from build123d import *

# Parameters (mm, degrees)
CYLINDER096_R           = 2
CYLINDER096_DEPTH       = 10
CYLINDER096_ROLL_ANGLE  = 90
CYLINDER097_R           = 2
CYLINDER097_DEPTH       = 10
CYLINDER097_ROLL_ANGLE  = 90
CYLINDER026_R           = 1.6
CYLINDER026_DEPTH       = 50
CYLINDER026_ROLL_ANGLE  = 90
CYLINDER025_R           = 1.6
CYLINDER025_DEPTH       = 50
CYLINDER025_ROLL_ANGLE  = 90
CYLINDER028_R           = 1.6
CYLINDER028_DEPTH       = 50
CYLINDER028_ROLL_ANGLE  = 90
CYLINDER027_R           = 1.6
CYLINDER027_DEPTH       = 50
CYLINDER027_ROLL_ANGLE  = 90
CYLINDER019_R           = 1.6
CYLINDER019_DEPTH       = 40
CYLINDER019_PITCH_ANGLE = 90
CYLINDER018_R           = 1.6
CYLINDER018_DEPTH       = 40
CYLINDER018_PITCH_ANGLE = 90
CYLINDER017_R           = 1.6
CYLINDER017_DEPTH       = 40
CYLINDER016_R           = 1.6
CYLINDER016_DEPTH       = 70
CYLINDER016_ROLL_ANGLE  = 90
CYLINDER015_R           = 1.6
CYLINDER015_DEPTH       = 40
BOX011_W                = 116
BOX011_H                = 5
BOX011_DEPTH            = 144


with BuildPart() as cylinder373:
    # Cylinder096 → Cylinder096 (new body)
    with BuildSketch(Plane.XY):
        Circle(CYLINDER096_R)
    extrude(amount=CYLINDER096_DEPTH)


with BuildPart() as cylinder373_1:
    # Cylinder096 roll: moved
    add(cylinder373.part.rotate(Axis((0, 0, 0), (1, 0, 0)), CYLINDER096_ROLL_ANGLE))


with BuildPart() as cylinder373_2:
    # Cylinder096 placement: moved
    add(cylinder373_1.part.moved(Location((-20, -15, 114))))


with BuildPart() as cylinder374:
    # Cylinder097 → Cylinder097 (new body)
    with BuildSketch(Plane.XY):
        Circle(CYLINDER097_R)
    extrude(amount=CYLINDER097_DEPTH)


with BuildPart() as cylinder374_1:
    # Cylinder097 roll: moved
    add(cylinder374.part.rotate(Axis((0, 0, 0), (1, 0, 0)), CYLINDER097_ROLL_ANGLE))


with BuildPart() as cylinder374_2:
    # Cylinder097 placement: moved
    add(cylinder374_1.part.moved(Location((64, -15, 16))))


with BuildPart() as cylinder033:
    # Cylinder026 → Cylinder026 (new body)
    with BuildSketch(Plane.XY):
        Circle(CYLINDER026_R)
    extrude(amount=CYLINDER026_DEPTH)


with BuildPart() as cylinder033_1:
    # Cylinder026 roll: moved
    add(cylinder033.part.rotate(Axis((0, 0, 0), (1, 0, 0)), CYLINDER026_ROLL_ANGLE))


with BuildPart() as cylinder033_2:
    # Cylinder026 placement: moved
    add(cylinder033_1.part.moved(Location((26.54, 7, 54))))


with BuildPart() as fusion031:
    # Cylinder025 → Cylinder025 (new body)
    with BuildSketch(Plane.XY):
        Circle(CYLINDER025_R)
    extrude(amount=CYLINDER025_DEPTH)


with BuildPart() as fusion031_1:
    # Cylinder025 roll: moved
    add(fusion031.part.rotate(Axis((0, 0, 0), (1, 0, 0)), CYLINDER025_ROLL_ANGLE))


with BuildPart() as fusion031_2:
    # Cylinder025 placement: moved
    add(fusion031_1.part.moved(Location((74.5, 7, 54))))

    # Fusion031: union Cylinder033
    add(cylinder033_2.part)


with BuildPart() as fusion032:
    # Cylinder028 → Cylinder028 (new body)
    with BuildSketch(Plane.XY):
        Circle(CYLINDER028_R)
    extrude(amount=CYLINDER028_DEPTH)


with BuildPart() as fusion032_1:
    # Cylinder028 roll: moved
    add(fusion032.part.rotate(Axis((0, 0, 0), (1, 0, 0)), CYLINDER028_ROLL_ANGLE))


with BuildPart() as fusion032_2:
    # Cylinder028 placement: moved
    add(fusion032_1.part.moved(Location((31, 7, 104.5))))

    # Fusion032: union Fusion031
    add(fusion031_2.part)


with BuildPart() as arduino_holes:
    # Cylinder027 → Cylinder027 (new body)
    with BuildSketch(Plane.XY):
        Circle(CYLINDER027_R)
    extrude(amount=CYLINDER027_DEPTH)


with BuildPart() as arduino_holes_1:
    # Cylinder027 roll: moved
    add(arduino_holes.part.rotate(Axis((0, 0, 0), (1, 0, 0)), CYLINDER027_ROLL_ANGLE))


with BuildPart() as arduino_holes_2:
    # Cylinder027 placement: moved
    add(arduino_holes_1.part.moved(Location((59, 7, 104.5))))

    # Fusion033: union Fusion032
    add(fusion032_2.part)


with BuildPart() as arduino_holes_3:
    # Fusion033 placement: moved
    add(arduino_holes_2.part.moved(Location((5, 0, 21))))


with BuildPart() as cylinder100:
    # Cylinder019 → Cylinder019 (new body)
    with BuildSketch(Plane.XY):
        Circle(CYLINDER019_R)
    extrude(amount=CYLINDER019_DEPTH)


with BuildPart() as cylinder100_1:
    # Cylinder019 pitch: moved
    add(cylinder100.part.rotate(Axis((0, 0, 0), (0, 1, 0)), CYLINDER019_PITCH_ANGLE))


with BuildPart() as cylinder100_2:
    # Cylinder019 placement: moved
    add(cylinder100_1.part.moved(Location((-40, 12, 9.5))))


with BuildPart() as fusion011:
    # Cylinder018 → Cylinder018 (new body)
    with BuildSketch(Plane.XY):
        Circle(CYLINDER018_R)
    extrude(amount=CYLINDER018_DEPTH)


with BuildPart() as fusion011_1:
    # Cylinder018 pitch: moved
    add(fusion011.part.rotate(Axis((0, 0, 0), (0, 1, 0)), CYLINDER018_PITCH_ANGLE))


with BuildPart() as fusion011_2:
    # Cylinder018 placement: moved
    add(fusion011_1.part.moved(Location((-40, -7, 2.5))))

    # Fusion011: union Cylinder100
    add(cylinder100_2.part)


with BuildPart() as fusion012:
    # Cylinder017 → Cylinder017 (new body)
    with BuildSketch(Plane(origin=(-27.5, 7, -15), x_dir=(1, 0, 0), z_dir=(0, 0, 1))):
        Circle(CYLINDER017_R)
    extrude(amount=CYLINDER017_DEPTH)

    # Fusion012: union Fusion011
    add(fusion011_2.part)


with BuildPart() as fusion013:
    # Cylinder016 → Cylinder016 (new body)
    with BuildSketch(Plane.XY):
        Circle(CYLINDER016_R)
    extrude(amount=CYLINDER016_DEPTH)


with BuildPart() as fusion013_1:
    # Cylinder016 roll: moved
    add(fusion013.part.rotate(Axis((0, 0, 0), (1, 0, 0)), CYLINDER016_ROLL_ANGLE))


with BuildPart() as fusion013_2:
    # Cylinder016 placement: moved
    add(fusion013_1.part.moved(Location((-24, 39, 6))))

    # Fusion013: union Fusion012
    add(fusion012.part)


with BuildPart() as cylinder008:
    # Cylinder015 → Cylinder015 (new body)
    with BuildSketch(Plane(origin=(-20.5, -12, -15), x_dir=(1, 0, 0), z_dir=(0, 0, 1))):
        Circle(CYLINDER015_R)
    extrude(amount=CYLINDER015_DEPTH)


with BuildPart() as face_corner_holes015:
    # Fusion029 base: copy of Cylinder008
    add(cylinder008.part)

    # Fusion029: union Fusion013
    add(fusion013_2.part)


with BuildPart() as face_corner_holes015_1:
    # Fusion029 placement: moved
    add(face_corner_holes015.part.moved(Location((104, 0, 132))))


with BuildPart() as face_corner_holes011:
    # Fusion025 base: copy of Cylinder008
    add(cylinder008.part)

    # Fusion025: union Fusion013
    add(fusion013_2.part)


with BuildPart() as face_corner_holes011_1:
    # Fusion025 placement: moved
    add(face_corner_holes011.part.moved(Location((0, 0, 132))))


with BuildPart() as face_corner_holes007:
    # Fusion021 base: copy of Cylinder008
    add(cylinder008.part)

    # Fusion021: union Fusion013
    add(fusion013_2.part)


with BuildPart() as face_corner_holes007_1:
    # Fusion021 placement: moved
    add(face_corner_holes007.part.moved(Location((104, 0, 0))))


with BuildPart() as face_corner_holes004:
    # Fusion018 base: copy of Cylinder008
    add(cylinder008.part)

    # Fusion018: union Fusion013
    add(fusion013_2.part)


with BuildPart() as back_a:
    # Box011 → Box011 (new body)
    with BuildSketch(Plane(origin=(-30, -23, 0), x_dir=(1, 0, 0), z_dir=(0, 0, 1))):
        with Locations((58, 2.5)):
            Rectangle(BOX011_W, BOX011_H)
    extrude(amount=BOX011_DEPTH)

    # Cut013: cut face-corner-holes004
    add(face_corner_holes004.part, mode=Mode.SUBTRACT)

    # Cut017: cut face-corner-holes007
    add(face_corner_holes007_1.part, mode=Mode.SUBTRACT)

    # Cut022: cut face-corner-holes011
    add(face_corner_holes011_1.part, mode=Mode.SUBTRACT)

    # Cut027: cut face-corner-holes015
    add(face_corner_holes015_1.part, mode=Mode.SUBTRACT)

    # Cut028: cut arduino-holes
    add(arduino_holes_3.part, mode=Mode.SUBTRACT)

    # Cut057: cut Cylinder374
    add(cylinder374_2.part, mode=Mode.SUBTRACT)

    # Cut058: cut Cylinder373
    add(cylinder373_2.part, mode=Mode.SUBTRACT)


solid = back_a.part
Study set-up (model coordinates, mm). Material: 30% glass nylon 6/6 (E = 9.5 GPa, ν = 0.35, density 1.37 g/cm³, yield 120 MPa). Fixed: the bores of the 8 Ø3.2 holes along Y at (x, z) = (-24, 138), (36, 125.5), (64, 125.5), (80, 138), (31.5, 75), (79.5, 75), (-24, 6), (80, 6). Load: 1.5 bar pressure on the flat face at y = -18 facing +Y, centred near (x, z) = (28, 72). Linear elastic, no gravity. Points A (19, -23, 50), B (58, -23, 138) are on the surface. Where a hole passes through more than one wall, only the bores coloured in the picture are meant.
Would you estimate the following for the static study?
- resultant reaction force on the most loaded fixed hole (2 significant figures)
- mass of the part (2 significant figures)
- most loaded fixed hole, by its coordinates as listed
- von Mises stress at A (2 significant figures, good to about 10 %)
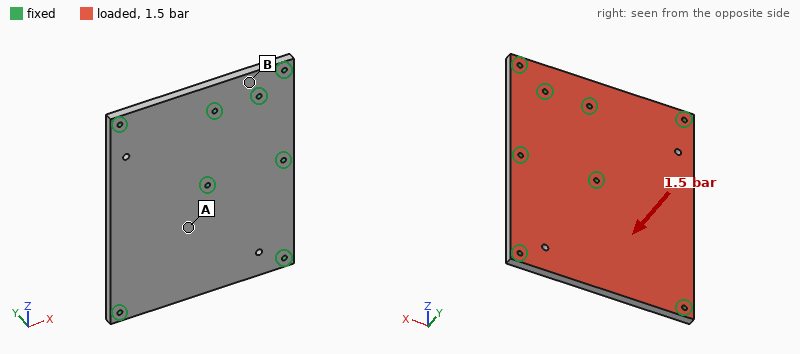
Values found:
850 N
110 g
(31.5, 75)
13 MPa
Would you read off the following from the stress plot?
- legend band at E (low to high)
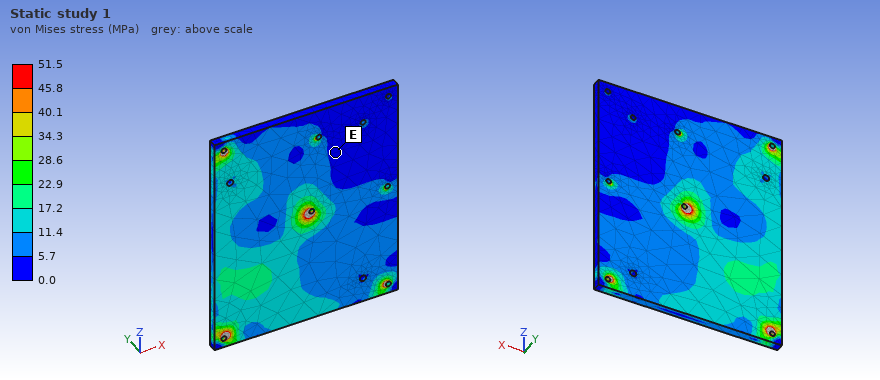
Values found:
0.0 to 5.7 MPa
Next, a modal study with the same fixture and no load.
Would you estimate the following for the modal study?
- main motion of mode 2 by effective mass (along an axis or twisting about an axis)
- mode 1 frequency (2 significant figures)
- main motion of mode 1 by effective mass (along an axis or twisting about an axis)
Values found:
along Y
1000 Hz
along Y
